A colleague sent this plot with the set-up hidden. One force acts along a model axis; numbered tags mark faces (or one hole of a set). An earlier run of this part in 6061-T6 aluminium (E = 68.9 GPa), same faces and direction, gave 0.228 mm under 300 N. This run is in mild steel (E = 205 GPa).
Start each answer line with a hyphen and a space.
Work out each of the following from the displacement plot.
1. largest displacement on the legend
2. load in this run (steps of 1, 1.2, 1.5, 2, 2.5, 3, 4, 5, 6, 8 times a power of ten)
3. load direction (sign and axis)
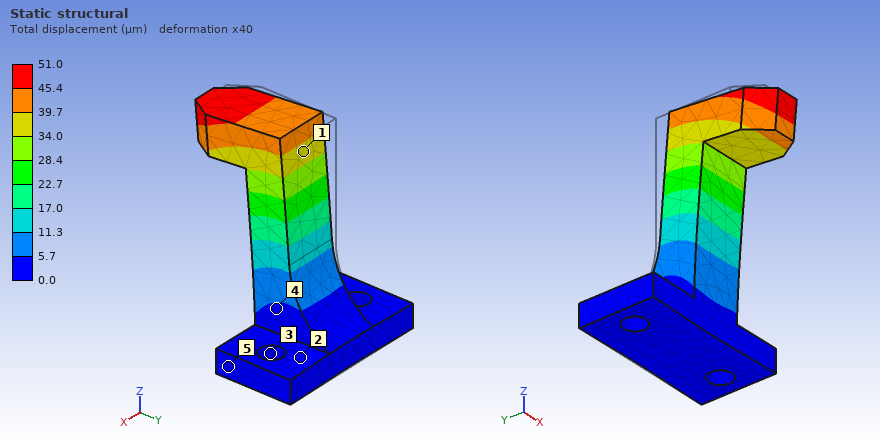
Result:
- 51.0 µm
- 200 N
- -Y
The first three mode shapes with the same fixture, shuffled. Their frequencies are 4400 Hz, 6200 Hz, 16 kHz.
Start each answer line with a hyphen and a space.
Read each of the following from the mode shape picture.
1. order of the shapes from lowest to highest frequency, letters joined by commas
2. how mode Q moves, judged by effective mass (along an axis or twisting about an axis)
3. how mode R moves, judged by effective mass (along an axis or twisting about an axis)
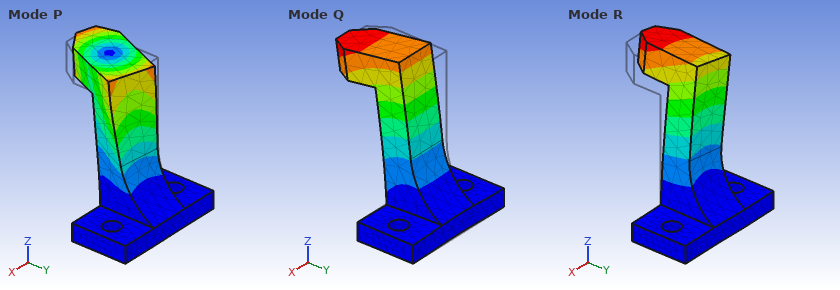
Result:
- Q, R, P
- along Y
- along X
